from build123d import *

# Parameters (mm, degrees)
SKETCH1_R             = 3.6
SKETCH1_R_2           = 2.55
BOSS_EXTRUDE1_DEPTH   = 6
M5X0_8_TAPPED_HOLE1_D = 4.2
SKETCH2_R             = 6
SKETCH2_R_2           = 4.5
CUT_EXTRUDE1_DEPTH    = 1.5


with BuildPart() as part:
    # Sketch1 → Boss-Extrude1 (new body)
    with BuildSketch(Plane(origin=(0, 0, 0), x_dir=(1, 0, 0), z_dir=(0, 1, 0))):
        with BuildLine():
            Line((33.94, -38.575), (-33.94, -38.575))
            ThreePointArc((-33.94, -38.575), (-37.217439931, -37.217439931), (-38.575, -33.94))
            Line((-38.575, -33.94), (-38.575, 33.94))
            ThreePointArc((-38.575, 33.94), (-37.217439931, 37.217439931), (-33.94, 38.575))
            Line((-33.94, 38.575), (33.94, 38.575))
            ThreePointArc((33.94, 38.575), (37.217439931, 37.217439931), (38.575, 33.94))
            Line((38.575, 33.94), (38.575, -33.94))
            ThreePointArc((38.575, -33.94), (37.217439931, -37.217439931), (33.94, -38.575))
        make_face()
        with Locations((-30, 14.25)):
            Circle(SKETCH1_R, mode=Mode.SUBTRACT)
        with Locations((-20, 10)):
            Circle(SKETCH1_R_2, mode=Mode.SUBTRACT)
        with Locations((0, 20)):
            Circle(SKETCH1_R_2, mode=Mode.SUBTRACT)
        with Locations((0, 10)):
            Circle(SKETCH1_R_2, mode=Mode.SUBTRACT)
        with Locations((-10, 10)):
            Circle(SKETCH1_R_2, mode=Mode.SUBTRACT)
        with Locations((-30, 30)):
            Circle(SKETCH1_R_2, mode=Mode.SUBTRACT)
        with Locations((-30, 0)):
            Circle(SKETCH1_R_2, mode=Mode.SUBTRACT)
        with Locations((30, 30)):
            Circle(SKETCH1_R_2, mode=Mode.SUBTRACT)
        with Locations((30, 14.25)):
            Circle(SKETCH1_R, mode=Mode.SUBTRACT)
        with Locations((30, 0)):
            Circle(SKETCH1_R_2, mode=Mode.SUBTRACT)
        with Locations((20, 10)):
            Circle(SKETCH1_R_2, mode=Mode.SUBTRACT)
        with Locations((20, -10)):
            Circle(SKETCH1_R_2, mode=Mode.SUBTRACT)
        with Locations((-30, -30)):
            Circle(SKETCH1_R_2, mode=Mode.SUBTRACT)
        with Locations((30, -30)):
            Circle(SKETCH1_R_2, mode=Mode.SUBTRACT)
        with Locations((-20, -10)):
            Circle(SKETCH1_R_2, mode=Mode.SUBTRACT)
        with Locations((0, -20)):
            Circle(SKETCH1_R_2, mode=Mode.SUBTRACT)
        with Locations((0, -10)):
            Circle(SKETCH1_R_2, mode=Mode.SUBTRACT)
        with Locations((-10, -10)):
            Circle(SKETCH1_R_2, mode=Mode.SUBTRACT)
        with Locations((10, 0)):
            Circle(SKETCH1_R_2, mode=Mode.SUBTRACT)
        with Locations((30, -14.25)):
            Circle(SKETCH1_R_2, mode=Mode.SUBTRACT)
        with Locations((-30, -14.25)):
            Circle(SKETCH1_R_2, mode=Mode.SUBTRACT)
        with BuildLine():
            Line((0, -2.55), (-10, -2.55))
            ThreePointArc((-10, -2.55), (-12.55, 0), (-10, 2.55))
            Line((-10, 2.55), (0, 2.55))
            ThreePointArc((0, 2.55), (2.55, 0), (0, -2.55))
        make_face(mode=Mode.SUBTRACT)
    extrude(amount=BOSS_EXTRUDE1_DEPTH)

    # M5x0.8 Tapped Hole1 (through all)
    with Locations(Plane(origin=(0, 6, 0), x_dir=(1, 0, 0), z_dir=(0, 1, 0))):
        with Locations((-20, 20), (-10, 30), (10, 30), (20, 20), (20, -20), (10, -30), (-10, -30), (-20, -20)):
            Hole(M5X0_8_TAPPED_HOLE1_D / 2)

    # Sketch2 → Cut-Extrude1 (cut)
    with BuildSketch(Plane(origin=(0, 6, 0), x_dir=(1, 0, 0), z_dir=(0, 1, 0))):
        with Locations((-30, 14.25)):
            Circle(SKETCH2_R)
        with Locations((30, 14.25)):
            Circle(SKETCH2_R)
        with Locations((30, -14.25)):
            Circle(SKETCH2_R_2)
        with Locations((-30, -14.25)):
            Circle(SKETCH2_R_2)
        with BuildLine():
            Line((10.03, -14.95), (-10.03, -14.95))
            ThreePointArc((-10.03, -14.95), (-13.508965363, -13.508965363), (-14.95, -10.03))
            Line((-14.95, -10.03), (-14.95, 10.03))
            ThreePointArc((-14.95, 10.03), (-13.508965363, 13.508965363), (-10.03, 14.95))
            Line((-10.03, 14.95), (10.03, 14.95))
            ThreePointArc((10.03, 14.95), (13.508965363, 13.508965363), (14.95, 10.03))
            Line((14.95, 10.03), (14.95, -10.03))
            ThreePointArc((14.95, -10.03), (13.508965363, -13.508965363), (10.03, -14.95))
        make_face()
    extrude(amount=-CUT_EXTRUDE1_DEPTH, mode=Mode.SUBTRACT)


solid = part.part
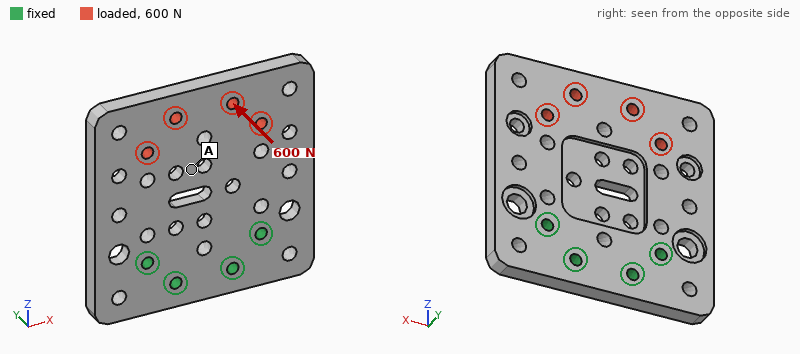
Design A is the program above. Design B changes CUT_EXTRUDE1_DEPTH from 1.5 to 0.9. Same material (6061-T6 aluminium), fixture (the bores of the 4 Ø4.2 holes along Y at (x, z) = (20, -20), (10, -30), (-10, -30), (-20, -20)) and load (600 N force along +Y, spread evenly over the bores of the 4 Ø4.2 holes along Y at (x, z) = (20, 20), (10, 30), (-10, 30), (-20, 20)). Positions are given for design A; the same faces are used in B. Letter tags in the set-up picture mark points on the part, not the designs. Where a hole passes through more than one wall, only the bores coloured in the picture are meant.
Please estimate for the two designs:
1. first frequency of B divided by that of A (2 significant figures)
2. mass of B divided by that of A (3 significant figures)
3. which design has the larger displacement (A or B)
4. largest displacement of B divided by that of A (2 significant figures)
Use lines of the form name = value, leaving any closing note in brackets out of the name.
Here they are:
first frequency of B divided by that of A = 1.0
mass of B divided by that of A = 1.02
which design has the larger displacement = A
largest displacement of B divided by that of A = 0.92
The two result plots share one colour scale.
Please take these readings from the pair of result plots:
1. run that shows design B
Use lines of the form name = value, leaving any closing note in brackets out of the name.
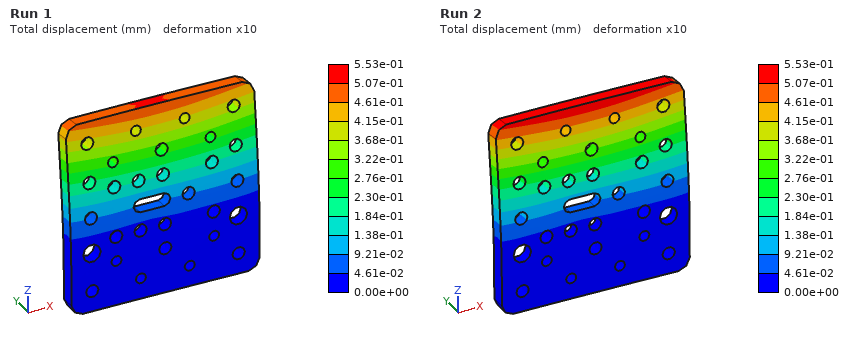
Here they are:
run that shows design B = Run 1
